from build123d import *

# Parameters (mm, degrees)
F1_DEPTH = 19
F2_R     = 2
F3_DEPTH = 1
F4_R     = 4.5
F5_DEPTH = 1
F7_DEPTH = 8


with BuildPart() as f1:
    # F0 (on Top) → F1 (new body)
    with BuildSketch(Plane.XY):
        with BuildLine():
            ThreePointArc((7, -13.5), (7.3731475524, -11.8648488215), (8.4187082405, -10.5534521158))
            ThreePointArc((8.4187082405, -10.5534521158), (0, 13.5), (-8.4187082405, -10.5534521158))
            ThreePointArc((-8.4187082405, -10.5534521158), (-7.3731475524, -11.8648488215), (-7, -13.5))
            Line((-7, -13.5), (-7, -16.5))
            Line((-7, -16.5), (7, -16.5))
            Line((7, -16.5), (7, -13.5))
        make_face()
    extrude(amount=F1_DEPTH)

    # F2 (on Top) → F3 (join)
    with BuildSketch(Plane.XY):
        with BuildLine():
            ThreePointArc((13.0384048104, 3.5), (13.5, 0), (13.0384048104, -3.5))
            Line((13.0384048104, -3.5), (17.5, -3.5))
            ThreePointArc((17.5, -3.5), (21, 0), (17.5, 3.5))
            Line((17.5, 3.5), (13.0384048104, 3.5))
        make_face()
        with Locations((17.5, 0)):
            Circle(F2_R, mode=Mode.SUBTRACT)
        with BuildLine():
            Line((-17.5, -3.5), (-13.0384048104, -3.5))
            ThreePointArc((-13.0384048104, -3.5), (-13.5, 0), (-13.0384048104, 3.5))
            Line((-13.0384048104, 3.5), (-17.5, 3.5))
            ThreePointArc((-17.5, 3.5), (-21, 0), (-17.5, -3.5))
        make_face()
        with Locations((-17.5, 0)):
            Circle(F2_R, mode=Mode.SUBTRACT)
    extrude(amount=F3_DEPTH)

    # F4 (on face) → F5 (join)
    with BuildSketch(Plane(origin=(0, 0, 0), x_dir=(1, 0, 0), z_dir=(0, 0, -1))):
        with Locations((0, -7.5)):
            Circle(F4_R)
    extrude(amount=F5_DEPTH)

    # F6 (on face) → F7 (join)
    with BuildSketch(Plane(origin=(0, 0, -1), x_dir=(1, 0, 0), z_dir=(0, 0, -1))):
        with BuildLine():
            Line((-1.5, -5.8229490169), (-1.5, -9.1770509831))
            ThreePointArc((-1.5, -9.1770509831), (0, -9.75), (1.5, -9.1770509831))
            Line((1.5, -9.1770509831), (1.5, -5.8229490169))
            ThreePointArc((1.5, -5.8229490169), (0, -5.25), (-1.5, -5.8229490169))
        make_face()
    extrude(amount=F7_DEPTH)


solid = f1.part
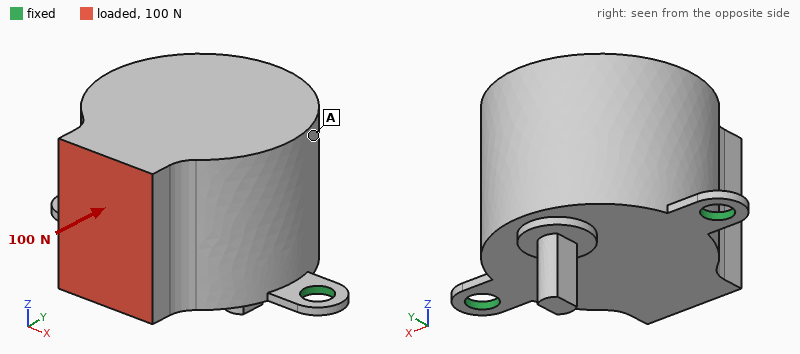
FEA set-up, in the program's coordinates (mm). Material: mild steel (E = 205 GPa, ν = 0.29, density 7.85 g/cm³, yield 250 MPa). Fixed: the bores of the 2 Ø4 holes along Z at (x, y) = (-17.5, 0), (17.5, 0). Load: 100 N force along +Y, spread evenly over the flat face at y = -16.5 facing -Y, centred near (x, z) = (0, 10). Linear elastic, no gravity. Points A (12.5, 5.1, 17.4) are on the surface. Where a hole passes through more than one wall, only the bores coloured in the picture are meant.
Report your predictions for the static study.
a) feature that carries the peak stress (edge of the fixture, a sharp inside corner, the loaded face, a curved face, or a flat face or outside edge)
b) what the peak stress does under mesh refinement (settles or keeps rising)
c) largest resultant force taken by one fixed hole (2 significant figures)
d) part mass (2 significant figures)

edge of the fixture
keeps rising
50 N
95 g
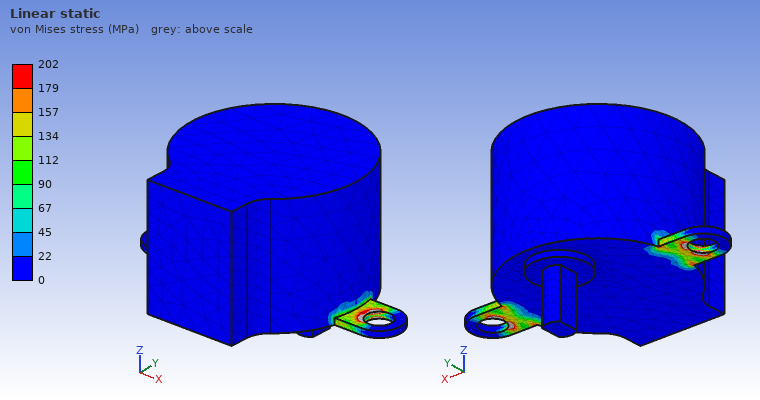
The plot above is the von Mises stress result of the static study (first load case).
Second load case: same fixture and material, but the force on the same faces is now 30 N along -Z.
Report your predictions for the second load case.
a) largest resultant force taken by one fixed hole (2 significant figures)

18 N
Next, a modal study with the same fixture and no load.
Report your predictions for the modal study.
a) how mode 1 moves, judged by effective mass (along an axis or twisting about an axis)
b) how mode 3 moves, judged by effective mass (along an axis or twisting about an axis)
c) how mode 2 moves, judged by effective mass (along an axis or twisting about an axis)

along Y
along X
along Z
